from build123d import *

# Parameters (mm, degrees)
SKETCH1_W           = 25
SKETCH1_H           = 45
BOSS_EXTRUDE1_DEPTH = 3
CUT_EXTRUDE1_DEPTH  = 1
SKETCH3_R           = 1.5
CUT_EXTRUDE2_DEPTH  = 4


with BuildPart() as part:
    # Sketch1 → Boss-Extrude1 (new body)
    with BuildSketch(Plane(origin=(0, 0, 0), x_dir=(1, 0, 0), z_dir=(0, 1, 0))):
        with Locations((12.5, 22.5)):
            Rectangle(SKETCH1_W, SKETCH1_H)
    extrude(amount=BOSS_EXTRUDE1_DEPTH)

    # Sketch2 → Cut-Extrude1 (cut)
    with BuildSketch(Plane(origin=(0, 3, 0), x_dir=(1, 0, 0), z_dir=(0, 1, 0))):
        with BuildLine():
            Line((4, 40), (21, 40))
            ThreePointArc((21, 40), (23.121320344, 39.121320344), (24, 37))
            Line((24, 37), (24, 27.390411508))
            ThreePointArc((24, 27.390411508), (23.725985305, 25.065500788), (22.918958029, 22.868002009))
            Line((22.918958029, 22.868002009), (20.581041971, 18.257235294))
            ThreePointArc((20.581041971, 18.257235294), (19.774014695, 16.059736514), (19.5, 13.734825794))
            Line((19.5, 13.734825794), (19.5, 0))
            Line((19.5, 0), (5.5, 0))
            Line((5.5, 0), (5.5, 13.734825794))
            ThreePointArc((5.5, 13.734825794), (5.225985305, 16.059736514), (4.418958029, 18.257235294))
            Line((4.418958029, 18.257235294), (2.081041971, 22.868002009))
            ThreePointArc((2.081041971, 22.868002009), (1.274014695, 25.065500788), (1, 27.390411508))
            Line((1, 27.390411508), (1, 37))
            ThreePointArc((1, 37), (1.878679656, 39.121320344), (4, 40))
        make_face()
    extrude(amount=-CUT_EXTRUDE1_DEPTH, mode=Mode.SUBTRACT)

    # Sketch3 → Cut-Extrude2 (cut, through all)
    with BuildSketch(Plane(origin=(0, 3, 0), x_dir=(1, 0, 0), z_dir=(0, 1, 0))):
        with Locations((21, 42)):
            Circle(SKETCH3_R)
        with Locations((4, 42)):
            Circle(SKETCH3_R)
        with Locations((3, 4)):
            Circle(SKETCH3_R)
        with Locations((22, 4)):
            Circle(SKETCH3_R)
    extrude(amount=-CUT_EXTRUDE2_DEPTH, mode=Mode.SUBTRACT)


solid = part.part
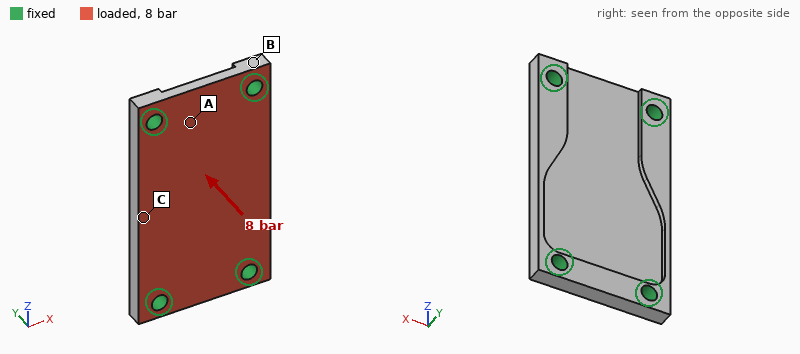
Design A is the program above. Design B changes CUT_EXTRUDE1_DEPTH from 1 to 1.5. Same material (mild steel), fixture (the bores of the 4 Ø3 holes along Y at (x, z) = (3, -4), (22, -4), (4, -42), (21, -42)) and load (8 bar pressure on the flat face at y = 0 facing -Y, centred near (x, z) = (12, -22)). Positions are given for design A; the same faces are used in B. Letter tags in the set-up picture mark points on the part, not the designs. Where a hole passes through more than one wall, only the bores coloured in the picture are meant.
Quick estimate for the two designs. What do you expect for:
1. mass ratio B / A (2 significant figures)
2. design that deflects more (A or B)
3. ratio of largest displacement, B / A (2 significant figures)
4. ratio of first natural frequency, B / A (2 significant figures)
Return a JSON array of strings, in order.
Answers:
["0.86", "B", "1.5", "0.95"]
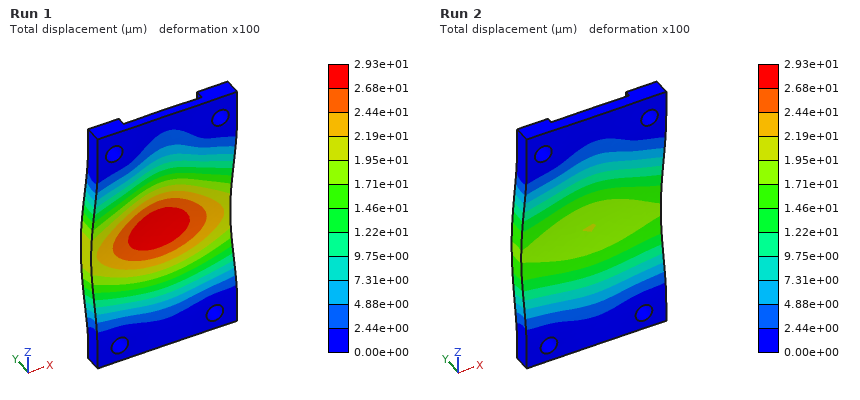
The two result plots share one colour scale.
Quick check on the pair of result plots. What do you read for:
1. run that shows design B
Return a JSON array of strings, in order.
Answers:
["Run 1"]
